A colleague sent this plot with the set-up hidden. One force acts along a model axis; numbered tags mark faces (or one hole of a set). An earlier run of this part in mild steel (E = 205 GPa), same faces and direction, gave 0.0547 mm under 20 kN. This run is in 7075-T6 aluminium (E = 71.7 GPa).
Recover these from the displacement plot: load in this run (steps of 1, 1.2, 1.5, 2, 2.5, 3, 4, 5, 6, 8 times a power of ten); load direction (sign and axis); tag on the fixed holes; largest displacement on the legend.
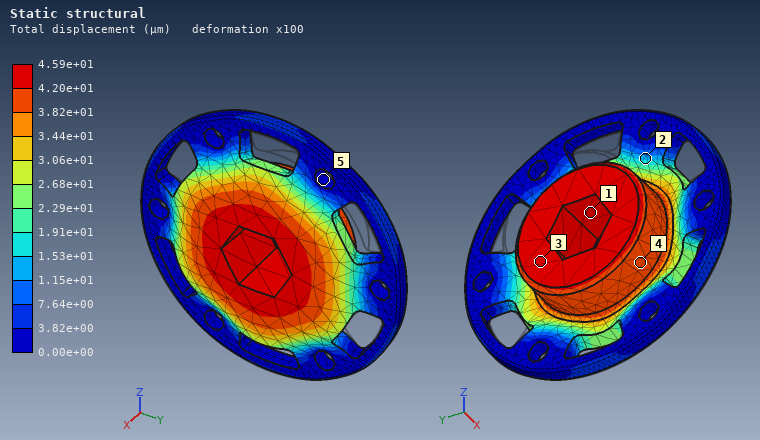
6 kN
+X
5
4.59e+01 µm
